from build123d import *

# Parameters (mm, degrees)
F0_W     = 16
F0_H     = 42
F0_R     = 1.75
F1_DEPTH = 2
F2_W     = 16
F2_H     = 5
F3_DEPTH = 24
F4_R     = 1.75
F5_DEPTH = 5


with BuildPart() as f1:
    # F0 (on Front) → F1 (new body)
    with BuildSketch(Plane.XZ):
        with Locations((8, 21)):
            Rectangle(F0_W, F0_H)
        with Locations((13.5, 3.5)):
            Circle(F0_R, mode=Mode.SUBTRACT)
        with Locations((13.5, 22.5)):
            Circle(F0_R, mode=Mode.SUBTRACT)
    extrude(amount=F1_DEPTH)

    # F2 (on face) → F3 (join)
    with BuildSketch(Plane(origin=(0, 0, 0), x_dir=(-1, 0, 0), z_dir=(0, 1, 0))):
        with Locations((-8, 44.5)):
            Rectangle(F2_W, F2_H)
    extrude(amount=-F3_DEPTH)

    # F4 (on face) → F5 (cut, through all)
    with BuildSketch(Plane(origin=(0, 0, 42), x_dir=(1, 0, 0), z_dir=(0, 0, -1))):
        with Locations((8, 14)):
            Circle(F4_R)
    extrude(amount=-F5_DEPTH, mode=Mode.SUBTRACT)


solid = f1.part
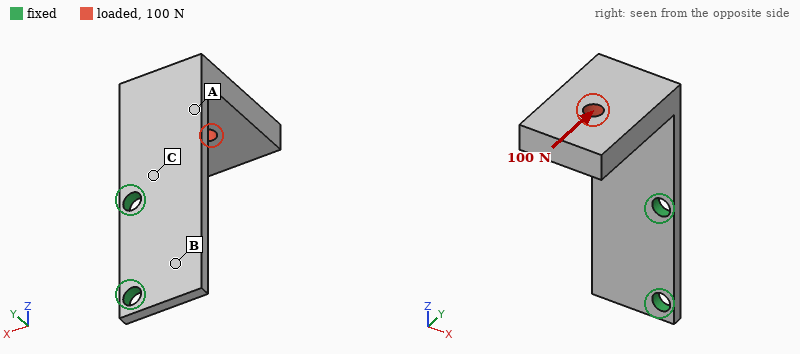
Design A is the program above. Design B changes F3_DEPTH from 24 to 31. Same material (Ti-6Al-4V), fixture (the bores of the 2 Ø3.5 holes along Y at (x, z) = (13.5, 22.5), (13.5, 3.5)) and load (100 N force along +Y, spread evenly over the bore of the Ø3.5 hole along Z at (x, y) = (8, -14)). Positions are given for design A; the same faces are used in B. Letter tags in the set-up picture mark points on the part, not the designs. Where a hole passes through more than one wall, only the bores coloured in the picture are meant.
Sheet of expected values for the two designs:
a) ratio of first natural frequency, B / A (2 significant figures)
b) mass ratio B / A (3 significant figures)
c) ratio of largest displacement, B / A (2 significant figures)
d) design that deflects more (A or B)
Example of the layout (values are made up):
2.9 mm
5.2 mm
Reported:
0.76
1.18
1.2
B
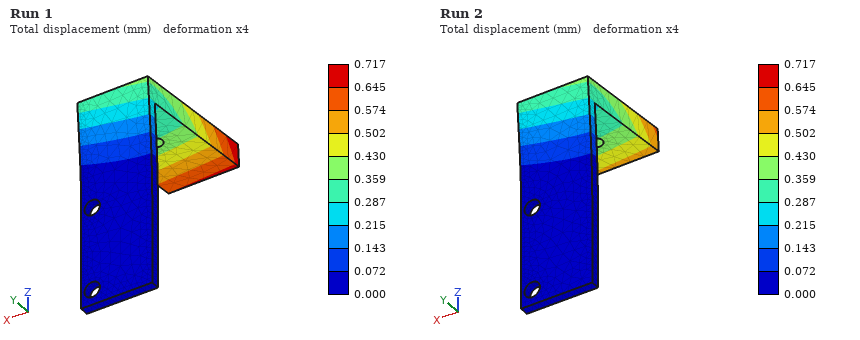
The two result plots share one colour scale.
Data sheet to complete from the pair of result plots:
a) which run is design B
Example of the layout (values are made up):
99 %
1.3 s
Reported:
Run 1
